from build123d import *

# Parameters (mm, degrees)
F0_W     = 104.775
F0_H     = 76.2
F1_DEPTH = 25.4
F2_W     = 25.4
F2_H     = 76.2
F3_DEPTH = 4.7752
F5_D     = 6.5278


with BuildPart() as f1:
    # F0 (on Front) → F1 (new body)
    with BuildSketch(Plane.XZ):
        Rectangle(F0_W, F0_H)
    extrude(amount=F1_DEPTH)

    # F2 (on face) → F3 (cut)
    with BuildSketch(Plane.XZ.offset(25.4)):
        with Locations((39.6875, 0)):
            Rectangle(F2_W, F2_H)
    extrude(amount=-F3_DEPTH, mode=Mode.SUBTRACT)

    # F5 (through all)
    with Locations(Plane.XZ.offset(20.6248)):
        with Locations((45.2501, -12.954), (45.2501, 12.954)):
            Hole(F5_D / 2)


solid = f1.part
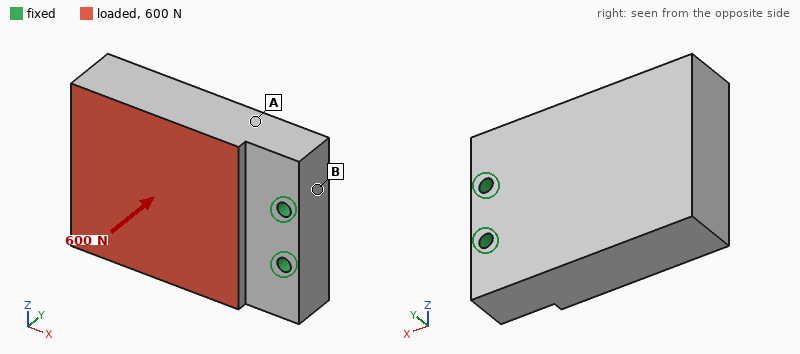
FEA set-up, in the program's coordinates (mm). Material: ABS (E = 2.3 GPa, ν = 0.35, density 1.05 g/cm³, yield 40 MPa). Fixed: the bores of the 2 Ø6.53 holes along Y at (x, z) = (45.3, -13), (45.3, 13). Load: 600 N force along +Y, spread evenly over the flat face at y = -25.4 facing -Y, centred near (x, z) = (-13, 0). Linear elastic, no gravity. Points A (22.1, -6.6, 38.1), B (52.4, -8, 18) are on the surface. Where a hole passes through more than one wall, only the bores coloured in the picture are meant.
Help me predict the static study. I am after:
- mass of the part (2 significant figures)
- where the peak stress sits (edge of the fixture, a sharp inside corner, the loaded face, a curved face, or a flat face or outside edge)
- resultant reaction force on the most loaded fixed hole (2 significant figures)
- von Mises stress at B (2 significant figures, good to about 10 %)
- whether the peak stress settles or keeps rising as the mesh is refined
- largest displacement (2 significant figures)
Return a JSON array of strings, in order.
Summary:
["200 g", "edge of the fixture", "300 N", "4.3 MPa", "keeps rising", "0.77 mm"]
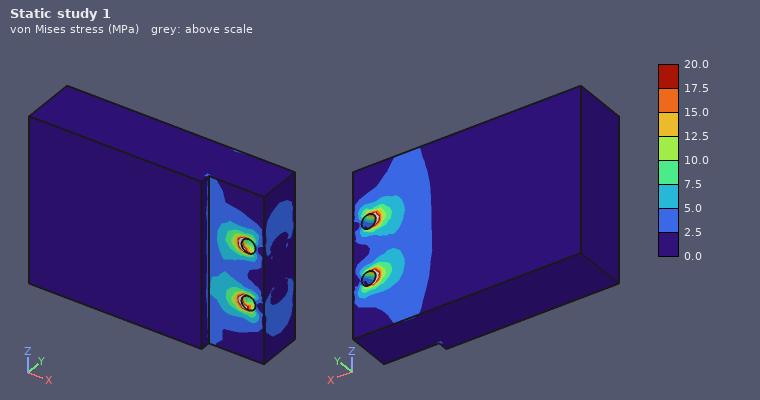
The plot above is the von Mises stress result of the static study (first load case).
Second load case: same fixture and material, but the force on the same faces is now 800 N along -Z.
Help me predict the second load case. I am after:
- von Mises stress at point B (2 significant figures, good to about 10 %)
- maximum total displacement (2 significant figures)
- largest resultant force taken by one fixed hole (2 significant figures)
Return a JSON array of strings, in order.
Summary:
["3.6 MPa", "0.33 mm", "1.5 kN"]
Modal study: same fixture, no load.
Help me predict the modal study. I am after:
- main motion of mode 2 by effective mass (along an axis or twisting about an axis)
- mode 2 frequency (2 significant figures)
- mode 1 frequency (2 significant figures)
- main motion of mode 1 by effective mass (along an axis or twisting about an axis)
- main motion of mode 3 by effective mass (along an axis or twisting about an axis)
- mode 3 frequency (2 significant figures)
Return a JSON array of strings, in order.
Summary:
["along Z", "770 Hz", "430 Hz", "along Y", "twisting about X", "1200 Hz"]
